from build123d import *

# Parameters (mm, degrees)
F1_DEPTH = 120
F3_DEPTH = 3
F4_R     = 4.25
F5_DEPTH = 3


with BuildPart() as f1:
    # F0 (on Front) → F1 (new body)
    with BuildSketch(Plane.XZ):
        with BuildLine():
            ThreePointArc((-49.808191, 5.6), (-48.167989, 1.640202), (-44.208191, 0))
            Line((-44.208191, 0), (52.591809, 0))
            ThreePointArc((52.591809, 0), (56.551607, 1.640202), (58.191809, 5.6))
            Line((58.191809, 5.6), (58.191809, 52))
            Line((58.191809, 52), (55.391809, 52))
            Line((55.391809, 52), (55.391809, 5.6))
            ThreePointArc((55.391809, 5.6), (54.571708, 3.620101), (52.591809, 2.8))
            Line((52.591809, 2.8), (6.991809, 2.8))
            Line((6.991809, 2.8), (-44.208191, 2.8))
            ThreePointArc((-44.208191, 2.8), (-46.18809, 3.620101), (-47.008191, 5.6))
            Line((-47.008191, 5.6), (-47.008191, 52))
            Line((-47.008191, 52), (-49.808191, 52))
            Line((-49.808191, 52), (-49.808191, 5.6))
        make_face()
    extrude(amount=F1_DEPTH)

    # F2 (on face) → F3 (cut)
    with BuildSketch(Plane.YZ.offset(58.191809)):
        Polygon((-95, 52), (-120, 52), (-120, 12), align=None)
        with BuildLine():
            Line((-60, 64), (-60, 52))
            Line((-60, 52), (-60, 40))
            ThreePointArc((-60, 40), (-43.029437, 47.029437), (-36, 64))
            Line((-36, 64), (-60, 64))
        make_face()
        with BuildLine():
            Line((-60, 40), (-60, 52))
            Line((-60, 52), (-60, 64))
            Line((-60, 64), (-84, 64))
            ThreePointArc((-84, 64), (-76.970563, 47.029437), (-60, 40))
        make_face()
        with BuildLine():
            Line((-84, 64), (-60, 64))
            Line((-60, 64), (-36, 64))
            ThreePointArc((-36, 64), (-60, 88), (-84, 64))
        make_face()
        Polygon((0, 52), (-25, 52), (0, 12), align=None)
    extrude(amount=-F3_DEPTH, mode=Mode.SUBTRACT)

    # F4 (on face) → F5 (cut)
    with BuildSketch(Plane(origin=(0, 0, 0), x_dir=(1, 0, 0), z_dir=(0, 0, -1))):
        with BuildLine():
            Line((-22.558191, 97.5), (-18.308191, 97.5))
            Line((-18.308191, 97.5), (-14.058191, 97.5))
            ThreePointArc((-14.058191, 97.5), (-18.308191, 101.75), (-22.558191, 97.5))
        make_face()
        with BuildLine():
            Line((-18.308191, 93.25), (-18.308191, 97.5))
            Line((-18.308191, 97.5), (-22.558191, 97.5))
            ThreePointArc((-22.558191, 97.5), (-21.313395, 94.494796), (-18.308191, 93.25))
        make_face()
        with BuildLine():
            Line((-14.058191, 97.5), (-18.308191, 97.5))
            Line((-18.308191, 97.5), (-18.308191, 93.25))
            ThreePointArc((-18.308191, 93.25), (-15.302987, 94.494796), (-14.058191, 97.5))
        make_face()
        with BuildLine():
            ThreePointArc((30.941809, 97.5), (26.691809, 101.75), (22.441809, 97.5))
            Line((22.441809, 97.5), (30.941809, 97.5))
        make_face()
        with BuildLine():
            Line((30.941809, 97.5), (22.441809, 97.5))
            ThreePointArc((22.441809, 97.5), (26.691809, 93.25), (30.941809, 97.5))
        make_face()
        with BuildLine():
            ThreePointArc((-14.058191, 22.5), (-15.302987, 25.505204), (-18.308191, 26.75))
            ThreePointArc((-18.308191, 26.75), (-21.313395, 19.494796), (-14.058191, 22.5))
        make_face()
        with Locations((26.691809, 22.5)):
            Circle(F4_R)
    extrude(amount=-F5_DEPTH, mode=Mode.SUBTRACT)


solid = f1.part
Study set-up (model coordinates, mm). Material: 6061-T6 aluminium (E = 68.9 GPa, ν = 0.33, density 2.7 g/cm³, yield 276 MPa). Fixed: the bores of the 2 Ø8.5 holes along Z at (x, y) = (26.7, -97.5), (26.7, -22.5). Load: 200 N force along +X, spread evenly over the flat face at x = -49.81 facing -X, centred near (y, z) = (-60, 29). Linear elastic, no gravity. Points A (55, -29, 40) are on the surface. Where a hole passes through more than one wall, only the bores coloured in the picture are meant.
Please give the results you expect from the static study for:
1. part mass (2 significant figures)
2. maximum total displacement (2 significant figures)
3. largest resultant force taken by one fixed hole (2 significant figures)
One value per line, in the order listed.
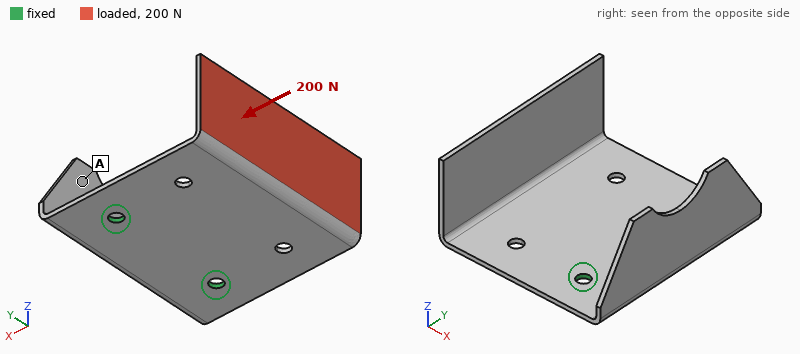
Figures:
170 g
1.8 mm
100 N
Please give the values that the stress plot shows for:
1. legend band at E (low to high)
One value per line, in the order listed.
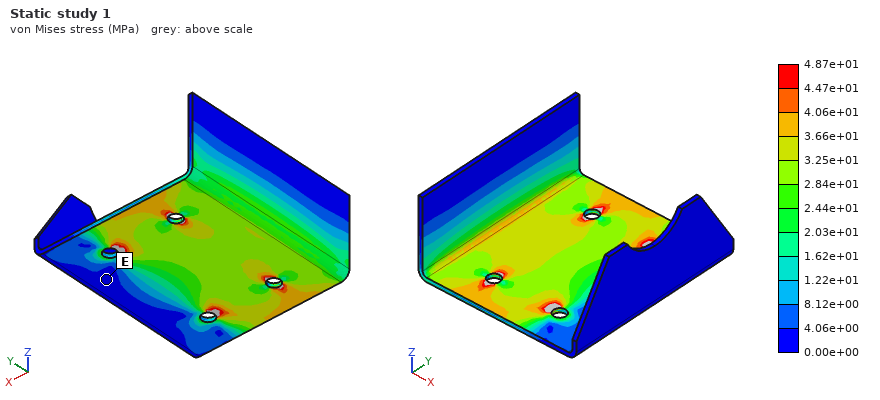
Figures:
0.00e+00 to 4.06e+00 MPa
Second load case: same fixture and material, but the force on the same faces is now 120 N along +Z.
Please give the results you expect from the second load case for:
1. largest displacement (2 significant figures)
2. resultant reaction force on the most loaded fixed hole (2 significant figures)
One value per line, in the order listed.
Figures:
1.6 mm
60 N
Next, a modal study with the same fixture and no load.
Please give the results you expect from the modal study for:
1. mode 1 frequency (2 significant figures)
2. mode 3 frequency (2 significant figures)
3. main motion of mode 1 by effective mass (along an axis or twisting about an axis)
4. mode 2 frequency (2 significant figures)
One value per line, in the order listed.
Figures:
190 Hz
590 Hz
along Z
360 Hz
